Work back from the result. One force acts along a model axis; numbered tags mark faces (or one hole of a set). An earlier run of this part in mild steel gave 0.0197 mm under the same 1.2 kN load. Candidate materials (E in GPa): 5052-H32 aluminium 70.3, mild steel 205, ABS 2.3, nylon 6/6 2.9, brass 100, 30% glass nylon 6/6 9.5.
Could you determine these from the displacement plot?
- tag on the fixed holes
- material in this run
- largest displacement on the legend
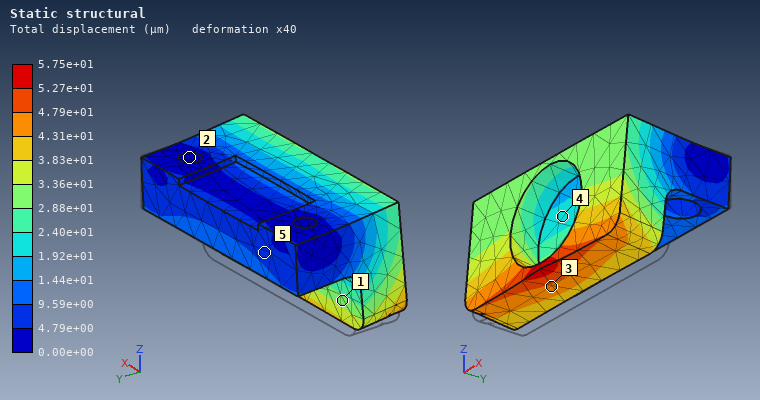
2
5052-H32 aluminium
5.75e+01 µm
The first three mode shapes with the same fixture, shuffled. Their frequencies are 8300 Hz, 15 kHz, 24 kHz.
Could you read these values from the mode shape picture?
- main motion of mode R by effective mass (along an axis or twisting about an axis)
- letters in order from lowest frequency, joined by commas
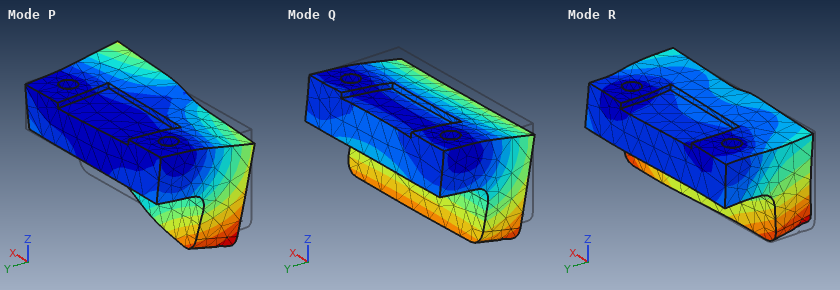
along X
Q, P, R
